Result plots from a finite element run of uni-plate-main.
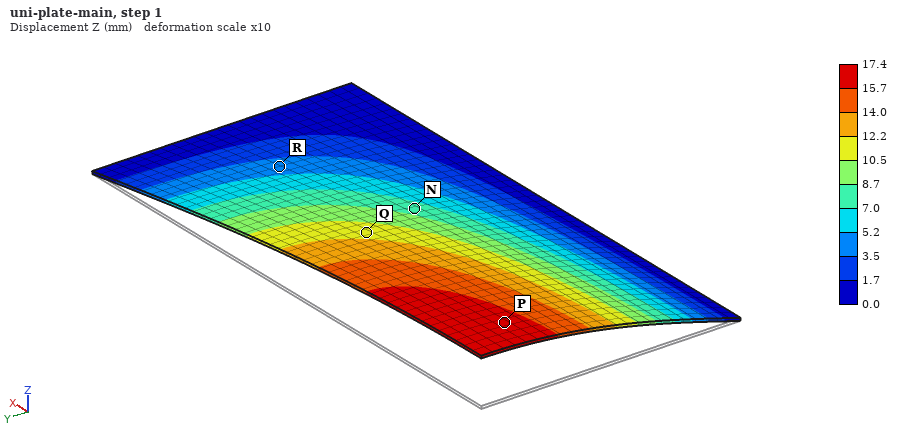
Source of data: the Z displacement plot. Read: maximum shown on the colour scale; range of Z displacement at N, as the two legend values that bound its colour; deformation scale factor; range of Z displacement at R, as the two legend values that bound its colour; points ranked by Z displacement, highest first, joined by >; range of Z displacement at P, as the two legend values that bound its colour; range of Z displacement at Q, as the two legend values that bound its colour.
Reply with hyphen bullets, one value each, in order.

- 17.4 mm
- 7.0 to 8.7 mm
- 10
- 3.5 to 5.2 mm
- P > Q > N > R
- 15.7 to 17.4 mm
- 10.5 to 12.2 mm
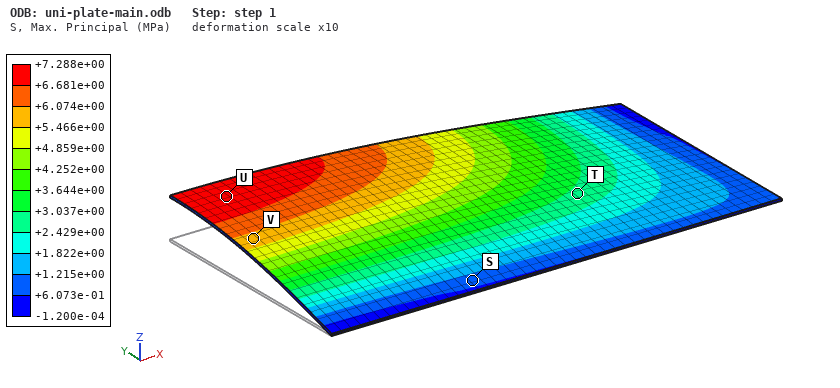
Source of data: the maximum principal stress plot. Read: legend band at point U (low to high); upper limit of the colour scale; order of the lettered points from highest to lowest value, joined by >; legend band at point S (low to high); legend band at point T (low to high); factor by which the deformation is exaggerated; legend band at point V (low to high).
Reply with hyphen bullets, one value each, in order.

- +6.681e+00 to +7.288e+00 MPa
- +7.288e+00 MPa
- U > V > T > S
- +6.073e-01 to +1.215e+00 MPa
- +2.429e+00 to +3.037e+00 MPa
- 10
- +5.466e+00 to +6.074e+00 MPa
